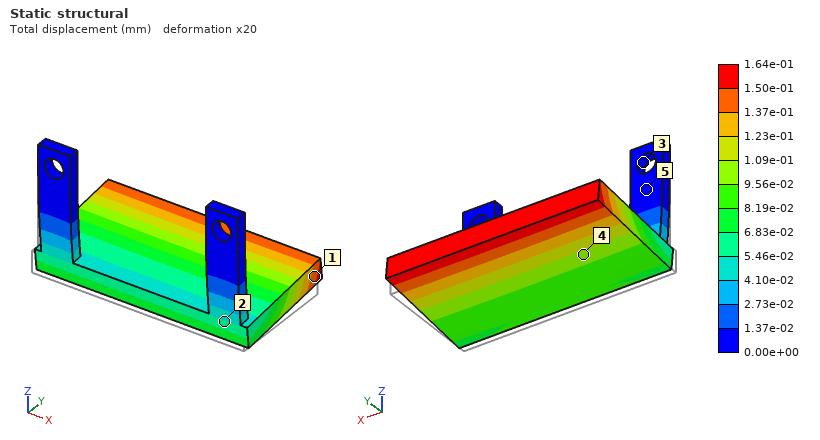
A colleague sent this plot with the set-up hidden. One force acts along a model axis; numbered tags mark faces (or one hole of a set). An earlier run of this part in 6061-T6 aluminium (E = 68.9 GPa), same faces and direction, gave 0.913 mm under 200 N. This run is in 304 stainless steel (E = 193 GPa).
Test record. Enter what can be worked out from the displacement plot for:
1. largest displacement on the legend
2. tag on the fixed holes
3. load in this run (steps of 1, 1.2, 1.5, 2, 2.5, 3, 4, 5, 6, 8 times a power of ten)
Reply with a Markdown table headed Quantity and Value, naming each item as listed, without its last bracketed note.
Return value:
| Quantity | Value |
|---|---|
| largest displacement on the legend | 1.64e-01 mm |
| tag on the fixed holes | 3 |
| load in this run | 100 N |
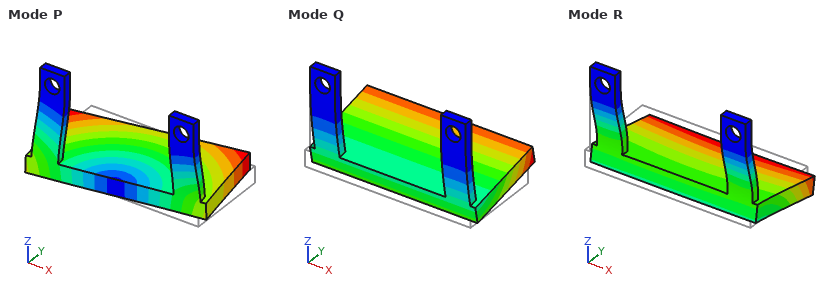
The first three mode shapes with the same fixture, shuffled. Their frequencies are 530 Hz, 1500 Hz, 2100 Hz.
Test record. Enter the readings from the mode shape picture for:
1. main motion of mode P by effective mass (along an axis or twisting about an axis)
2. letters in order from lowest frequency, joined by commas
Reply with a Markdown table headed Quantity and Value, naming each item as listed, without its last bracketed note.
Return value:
| Quantity | Value |
|---|---|
| main motion of mode P by effective mass | along X |
| letters in order from lowest frequency, joined by commas | Q, P, R |
